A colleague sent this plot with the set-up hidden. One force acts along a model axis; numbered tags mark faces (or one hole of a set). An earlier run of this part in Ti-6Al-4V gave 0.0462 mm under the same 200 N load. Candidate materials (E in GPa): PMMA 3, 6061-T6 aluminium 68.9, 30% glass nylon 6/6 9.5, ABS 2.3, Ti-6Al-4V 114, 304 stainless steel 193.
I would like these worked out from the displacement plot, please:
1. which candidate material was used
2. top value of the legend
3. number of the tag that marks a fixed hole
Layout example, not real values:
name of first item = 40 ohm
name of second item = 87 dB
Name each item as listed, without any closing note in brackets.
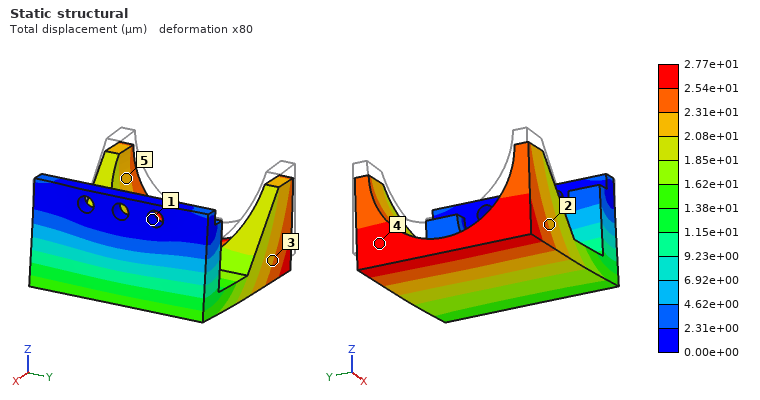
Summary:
which candidate material was used = 304 stainless steel
top value of the legend = 2.77e+01 µm
number of the tag that marks a fixed hole = 1
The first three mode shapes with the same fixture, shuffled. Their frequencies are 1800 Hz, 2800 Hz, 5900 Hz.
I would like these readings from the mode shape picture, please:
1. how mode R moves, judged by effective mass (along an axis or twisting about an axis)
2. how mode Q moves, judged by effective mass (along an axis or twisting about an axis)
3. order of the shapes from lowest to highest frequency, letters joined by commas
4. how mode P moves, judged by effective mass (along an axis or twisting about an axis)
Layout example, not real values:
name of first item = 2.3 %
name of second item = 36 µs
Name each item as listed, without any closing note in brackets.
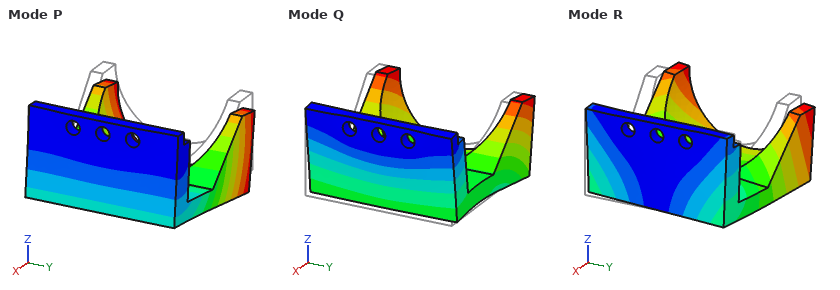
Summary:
how mode R moves, judged by effective mass = along Y
how mode Q moves, judged by effective mass = along X
order of the shapes from lowest to highest frequency, letters joined by commas = P, R, Q
how mode P moves, judged by effective mass = along Z
